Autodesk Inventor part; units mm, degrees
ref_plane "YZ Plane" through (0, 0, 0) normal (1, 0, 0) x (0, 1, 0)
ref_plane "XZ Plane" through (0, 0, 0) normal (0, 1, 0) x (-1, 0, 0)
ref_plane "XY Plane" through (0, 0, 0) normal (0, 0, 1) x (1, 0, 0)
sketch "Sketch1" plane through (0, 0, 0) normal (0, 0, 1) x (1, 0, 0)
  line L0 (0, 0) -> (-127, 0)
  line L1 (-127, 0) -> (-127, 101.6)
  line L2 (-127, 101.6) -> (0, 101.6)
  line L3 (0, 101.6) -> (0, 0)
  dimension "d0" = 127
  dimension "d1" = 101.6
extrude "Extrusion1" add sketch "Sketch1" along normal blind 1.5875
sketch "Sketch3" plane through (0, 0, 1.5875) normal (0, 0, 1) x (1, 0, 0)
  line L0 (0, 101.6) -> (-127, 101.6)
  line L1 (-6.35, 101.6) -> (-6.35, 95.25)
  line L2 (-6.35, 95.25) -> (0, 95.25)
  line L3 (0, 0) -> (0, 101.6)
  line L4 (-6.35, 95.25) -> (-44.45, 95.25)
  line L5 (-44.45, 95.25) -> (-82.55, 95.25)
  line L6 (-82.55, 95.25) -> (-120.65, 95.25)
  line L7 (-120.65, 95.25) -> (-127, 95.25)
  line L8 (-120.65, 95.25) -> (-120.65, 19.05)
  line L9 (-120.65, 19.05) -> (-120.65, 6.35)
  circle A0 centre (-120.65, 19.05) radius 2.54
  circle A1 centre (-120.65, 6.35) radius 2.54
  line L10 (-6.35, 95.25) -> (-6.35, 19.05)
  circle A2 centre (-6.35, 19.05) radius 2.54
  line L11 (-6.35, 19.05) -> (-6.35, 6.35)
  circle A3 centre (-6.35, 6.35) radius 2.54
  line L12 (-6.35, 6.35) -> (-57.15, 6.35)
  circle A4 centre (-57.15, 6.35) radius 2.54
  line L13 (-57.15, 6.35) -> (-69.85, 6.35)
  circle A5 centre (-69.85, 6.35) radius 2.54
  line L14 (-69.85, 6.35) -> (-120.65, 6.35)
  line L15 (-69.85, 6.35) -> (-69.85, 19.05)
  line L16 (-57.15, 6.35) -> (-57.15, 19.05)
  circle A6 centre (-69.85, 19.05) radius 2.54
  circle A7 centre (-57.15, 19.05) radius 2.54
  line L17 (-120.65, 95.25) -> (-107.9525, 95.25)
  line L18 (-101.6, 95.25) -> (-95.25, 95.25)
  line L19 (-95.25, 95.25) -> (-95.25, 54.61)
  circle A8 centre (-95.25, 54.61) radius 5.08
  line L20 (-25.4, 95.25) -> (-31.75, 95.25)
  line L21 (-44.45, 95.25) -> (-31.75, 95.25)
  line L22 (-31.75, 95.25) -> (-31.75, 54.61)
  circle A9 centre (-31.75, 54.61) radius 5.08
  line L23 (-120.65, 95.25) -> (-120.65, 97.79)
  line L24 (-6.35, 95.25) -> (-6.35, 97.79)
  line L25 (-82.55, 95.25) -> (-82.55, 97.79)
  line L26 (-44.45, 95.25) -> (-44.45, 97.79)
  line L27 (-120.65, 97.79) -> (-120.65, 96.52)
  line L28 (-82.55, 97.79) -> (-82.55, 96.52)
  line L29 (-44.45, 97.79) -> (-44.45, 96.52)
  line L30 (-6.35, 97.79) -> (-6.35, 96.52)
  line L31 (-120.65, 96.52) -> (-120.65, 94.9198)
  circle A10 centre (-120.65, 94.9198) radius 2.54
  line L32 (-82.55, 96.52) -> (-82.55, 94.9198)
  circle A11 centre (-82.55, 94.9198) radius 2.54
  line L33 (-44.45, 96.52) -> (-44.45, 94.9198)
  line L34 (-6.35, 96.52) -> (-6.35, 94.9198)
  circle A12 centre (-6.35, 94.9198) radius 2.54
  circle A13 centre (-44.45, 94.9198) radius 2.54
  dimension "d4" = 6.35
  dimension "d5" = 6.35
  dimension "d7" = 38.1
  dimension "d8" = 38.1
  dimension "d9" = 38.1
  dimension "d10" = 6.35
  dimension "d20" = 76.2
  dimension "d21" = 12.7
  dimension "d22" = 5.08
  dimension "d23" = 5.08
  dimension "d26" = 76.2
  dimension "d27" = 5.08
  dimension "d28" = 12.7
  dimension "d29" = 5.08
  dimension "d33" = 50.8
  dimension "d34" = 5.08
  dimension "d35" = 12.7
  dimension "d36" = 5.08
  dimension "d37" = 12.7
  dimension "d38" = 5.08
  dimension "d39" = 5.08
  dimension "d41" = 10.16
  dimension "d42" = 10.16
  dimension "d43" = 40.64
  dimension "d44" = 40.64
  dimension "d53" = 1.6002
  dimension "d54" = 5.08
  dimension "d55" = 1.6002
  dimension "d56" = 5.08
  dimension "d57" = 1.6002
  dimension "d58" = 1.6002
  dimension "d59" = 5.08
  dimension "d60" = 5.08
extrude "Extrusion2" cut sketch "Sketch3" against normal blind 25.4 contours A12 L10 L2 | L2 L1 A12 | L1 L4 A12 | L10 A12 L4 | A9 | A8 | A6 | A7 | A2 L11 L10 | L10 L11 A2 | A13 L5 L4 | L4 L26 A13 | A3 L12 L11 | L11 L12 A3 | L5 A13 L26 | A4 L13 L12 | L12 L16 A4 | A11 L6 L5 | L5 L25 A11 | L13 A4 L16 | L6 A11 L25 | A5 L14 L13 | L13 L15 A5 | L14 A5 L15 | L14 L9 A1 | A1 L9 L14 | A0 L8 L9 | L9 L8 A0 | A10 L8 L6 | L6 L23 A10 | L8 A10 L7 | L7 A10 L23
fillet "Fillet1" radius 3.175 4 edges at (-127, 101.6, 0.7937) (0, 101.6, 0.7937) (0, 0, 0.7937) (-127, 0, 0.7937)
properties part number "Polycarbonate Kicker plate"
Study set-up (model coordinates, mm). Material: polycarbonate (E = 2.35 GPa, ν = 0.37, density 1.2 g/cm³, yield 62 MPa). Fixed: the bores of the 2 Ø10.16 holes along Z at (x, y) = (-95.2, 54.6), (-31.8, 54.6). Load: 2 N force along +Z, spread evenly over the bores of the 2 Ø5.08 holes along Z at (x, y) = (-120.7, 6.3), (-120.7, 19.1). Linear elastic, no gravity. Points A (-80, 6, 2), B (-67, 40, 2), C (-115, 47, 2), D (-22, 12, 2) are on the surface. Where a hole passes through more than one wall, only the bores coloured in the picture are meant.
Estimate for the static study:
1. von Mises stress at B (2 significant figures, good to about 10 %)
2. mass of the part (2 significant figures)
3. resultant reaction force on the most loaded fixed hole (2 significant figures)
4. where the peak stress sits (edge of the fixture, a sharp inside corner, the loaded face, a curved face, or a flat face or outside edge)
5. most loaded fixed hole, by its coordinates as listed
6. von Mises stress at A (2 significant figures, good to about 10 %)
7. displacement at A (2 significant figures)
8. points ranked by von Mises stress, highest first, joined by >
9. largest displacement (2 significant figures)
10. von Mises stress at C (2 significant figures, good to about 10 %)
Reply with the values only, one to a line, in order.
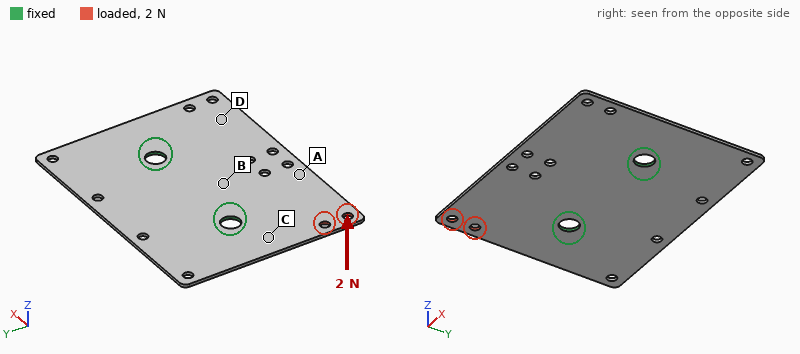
0.75 MPa
24 g
2.3 N
a flat face or outside edge
(-95.2, 54.6)
1.2 MPa
0.55 mm
C > A > B > D
1.9 mm
2.3 MPa
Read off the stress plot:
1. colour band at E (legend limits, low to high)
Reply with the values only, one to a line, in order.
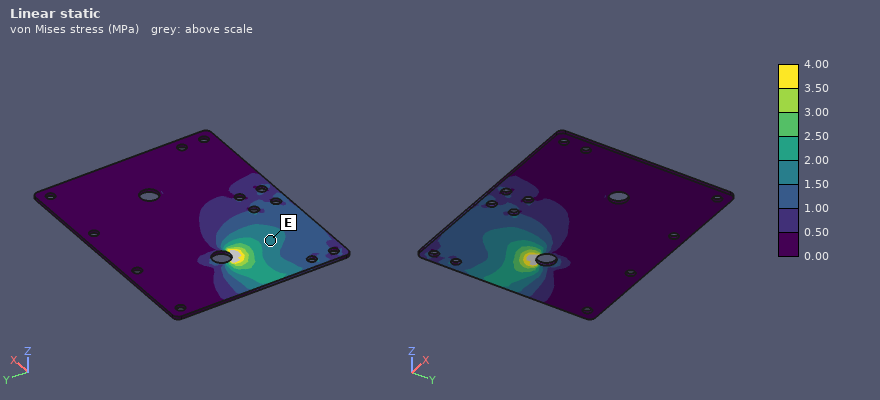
1.50 to 2.00 MPa
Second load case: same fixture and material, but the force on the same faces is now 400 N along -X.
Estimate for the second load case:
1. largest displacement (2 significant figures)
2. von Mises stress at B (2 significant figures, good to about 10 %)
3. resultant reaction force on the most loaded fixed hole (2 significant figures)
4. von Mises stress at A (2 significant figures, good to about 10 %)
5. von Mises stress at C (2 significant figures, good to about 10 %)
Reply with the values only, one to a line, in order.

0.44 mm
5.3 MPa
320 N
5.9 MPa
2.6 MPa
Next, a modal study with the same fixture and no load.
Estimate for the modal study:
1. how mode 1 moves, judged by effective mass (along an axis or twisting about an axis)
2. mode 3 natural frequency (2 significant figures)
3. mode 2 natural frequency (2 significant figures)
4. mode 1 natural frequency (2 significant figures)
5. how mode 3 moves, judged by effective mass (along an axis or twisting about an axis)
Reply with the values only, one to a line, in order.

along Z
180 Hz
170 Hz
130 Hz
along Z
